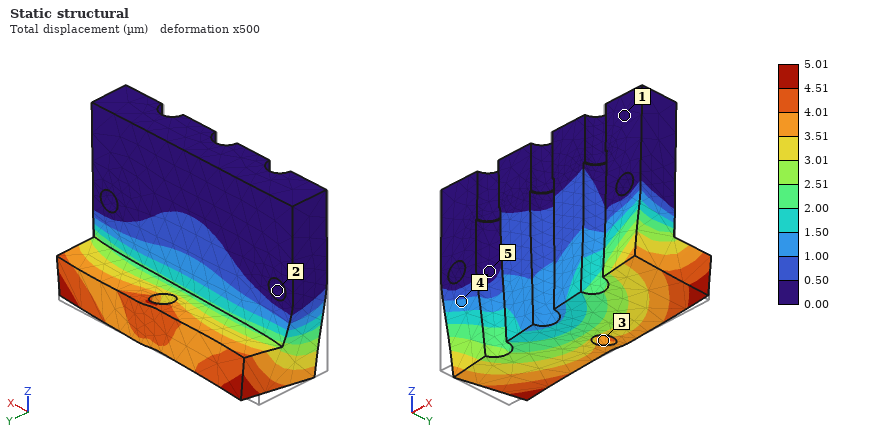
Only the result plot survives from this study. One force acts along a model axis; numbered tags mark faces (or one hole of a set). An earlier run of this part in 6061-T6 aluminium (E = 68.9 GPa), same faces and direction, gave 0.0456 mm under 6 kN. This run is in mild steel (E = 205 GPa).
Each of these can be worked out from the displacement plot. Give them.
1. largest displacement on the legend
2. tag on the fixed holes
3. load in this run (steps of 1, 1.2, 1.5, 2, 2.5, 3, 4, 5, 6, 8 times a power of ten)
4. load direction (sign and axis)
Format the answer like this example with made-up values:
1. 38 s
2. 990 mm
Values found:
1. 5.01 µm
2. 2
3. 2 kN
4. +X
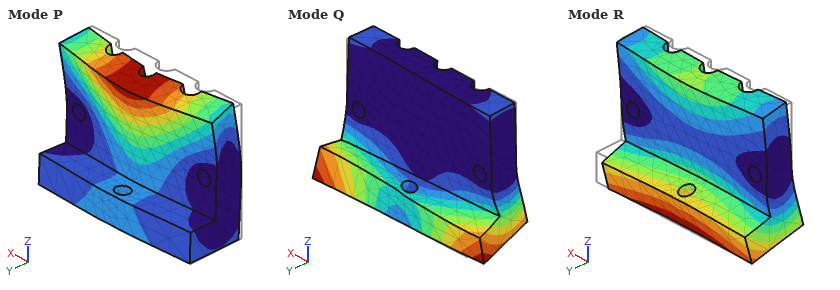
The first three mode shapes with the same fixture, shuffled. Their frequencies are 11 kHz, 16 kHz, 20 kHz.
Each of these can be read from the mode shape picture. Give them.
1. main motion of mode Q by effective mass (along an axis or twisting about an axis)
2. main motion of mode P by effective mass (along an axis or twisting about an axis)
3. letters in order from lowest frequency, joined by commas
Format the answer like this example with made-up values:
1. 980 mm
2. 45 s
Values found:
1. twisting about Z
2. along Y
3. R, P, Q
